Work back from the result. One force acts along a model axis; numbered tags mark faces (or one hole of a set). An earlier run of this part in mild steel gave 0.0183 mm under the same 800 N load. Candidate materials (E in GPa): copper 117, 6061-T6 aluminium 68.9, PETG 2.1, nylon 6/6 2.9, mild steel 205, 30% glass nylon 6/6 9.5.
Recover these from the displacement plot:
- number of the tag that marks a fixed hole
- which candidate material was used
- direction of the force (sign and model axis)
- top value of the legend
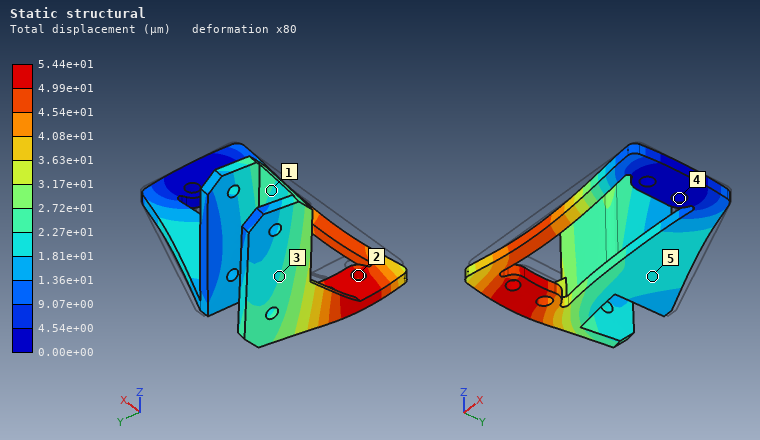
4
6061-T6 aluminium
-X
5.44e+01 µm
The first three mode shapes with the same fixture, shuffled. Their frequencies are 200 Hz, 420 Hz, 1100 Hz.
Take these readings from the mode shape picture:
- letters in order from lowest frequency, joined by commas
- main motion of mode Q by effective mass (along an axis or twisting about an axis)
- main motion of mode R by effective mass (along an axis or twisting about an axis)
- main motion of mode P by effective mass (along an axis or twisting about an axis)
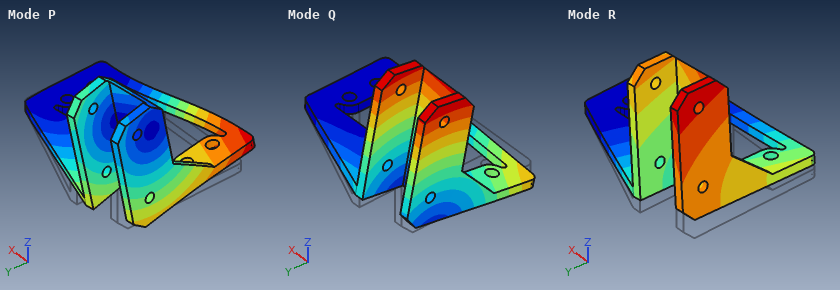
R, Q, P
along Y
along Z
along Y
